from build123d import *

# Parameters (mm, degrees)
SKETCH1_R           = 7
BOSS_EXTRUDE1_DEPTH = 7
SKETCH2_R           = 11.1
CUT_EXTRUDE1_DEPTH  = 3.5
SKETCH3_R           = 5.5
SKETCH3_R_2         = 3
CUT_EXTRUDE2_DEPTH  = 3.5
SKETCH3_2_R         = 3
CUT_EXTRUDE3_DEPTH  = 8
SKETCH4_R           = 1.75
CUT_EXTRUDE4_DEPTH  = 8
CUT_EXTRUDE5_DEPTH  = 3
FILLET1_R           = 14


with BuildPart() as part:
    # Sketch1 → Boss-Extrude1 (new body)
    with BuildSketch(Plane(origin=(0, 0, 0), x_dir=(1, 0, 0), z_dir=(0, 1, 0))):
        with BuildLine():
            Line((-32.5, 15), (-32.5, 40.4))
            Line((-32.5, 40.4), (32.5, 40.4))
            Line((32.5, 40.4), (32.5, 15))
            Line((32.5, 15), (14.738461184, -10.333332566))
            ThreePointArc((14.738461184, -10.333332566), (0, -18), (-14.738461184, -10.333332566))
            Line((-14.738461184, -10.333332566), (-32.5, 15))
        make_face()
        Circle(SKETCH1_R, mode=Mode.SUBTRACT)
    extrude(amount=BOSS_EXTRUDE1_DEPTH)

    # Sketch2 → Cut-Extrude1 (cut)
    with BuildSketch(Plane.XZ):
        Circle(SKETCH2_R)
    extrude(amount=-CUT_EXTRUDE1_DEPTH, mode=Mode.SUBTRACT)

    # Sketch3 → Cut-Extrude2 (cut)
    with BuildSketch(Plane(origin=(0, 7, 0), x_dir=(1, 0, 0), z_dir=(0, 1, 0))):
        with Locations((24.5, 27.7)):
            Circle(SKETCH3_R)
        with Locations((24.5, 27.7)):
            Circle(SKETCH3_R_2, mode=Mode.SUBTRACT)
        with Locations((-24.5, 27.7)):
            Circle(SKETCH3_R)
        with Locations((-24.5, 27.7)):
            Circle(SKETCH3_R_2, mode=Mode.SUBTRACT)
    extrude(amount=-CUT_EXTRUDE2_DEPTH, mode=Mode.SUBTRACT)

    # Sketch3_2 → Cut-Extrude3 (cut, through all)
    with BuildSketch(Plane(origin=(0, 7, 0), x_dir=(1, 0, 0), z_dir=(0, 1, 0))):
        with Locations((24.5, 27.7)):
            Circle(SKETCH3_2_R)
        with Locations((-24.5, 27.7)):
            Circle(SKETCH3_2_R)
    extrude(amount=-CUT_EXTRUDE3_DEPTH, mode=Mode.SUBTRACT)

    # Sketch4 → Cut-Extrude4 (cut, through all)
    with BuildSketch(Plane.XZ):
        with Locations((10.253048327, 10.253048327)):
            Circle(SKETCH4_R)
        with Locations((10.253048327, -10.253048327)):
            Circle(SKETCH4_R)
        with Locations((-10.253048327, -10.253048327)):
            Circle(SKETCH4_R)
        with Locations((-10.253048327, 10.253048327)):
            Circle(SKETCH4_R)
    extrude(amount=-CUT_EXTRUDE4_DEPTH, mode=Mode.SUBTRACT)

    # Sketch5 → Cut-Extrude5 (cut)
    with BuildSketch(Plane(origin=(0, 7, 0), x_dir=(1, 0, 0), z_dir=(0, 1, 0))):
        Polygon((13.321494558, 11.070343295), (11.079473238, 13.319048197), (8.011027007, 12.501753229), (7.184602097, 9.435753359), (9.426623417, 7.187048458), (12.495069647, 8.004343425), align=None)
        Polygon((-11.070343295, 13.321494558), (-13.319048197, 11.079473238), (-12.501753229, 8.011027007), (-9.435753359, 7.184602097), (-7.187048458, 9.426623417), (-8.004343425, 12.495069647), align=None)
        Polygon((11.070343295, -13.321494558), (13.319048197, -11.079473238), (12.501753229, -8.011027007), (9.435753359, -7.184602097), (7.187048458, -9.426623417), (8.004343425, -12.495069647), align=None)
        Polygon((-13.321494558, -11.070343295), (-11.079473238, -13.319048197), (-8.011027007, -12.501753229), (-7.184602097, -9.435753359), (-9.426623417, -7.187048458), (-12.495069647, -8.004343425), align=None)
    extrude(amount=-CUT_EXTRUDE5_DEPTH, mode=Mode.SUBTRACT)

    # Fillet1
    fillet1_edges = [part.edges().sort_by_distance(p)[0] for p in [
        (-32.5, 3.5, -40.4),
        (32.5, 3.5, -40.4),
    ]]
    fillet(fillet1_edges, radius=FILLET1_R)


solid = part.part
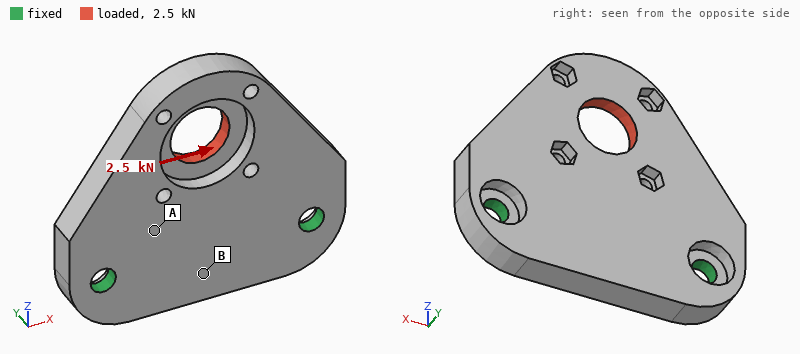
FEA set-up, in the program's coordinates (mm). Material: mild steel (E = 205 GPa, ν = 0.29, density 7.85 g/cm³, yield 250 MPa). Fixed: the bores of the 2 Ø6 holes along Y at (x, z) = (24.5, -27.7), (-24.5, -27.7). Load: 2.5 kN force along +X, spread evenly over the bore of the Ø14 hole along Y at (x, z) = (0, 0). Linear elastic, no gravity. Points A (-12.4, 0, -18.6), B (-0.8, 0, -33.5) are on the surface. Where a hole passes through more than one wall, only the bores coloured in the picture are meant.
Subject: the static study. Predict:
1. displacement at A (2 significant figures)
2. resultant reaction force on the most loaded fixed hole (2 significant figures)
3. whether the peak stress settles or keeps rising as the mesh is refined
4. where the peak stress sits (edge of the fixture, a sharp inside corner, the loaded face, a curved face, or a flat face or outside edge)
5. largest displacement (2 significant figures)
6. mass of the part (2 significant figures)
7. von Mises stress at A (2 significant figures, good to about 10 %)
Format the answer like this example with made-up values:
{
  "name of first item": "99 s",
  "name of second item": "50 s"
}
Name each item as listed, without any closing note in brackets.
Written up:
{
  "displacement at A": "1.4 µm",
  "resultant reaction force on the most loaded fixed hole": "1.8 kN",
  "whether the peak stress settles or keeps rising as the mesh is refined": "keeps rising",
  "where the peak stress sits": "edge of the fixture",
  "largest displacement": "7.3 µm",
  "mass of the part": "140 g",
  "von Mises stress at A": "14 MPa"
}
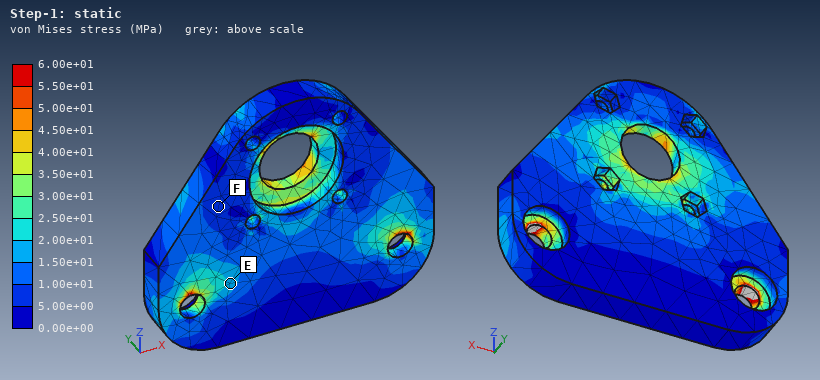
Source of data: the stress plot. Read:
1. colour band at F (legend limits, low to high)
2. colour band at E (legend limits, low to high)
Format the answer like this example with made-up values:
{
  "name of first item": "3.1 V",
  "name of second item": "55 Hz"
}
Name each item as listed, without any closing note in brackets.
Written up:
{
  "colour band at F": "5.00e+00 to 1.00e+01 MPa",
  "colour band at E": "1.50e+01 to 2.00e+01 MPa"
}
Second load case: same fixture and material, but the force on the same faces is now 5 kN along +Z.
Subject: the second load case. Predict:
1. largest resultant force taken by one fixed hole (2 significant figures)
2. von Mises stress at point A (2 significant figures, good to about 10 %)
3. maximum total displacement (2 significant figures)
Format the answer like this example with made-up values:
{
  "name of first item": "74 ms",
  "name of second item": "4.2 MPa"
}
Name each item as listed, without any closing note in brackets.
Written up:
{
  "largest resultant force taken by one fixed hole": "2.5 kN",
  "von Mises stress at point A": "17 MPa",
  "maximum total displacement": "71 µm"
}
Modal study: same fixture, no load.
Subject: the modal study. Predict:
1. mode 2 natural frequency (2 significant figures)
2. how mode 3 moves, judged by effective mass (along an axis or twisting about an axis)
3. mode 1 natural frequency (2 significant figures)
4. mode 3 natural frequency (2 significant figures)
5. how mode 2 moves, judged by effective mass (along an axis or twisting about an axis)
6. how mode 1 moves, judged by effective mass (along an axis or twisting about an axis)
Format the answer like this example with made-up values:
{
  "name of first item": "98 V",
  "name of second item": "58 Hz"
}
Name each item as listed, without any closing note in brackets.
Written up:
{
  "mode 2 natural frequency": "7900 Hz",
  "how mode 3 moves, judged by effective mass": "along Y",
  "mode 1 natural frequency": "2700 Hz",
  "mode 3 natural frequency": "10 kHz",
  "how mode 2 moves, judged by effective mass": "twisting about Z",
  "how mode 1 moves, judged by effective mass": "along Y"
}
